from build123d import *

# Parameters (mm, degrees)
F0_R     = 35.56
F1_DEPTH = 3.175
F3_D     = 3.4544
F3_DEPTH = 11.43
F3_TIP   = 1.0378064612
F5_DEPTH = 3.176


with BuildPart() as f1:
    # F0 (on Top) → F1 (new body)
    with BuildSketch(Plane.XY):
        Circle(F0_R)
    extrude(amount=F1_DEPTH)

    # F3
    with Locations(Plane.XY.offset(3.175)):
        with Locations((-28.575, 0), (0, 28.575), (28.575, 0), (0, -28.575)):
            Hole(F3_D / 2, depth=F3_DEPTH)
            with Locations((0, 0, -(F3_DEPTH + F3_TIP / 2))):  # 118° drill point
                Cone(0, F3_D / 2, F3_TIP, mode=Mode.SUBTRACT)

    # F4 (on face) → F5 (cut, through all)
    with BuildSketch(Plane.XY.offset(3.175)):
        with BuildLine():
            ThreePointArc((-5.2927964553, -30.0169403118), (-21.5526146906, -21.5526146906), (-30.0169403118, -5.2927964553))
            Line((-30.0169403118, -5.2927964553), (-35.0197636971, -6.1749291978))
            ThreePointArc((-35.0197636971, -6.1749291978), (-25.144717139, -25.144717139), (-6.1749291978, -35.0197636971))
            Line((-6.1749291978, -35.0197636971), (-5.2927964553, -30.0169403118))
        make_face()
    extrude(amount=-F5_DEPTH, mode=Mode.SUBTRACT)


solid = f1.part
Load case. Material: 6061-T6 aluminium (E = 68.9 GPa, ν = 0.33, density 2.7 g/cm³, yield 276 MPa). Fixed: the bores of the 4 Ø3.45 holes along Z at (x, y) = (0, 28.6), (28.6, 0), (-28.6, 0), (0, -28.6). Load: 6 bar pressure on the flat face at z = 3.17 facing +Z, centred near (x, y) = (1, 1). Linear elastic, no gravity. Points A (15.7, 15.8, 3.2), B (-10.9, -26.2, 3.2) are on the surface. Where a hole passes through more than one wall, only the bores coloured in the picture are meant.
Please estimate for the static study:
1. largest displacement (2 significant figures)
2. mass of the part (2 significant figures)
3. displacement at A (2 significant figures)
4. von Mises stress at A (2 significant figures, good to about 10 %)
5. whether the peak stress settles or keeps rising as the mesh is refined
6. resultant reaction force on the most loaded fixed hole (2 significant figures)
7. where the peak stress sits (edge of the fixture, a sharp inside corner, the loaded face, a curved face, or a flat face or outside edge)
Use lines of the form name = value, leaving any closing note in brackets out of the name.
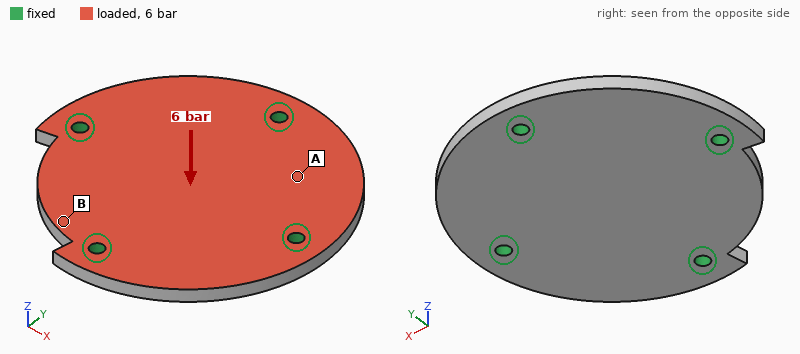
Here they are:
largest displacement = 49 µm
mass of the part = 32 g
displacement at A = 32 µm
von Mises stress at A = 31 MPa
whether the peak stress settles or keeps rising as the mesh is refined = keeps rising
resultant reaction force on the most loaded fixed hole = 600 N
where the peak stress sits = edge of the fixture
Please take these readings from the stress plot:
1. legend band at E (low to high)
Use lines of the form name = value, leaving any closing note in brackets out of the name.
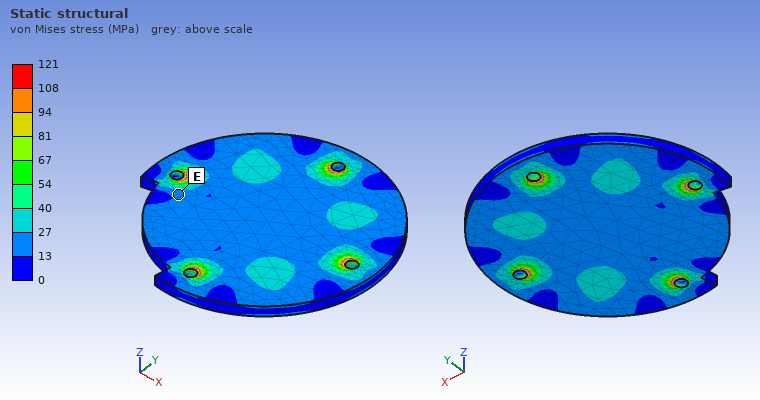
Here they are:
legend band at E = 13 to 27 MPa
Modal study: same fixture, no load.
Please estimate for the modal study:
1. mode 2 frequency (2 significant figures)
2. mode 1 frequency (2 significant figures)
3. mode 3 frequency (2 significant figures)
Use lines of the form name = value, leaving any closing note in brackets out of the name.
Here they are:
mode 2 frequency = 7300 Hz
mode 1 frequency = 7200 Hz
mode 3 frequency = 7700 Hz
